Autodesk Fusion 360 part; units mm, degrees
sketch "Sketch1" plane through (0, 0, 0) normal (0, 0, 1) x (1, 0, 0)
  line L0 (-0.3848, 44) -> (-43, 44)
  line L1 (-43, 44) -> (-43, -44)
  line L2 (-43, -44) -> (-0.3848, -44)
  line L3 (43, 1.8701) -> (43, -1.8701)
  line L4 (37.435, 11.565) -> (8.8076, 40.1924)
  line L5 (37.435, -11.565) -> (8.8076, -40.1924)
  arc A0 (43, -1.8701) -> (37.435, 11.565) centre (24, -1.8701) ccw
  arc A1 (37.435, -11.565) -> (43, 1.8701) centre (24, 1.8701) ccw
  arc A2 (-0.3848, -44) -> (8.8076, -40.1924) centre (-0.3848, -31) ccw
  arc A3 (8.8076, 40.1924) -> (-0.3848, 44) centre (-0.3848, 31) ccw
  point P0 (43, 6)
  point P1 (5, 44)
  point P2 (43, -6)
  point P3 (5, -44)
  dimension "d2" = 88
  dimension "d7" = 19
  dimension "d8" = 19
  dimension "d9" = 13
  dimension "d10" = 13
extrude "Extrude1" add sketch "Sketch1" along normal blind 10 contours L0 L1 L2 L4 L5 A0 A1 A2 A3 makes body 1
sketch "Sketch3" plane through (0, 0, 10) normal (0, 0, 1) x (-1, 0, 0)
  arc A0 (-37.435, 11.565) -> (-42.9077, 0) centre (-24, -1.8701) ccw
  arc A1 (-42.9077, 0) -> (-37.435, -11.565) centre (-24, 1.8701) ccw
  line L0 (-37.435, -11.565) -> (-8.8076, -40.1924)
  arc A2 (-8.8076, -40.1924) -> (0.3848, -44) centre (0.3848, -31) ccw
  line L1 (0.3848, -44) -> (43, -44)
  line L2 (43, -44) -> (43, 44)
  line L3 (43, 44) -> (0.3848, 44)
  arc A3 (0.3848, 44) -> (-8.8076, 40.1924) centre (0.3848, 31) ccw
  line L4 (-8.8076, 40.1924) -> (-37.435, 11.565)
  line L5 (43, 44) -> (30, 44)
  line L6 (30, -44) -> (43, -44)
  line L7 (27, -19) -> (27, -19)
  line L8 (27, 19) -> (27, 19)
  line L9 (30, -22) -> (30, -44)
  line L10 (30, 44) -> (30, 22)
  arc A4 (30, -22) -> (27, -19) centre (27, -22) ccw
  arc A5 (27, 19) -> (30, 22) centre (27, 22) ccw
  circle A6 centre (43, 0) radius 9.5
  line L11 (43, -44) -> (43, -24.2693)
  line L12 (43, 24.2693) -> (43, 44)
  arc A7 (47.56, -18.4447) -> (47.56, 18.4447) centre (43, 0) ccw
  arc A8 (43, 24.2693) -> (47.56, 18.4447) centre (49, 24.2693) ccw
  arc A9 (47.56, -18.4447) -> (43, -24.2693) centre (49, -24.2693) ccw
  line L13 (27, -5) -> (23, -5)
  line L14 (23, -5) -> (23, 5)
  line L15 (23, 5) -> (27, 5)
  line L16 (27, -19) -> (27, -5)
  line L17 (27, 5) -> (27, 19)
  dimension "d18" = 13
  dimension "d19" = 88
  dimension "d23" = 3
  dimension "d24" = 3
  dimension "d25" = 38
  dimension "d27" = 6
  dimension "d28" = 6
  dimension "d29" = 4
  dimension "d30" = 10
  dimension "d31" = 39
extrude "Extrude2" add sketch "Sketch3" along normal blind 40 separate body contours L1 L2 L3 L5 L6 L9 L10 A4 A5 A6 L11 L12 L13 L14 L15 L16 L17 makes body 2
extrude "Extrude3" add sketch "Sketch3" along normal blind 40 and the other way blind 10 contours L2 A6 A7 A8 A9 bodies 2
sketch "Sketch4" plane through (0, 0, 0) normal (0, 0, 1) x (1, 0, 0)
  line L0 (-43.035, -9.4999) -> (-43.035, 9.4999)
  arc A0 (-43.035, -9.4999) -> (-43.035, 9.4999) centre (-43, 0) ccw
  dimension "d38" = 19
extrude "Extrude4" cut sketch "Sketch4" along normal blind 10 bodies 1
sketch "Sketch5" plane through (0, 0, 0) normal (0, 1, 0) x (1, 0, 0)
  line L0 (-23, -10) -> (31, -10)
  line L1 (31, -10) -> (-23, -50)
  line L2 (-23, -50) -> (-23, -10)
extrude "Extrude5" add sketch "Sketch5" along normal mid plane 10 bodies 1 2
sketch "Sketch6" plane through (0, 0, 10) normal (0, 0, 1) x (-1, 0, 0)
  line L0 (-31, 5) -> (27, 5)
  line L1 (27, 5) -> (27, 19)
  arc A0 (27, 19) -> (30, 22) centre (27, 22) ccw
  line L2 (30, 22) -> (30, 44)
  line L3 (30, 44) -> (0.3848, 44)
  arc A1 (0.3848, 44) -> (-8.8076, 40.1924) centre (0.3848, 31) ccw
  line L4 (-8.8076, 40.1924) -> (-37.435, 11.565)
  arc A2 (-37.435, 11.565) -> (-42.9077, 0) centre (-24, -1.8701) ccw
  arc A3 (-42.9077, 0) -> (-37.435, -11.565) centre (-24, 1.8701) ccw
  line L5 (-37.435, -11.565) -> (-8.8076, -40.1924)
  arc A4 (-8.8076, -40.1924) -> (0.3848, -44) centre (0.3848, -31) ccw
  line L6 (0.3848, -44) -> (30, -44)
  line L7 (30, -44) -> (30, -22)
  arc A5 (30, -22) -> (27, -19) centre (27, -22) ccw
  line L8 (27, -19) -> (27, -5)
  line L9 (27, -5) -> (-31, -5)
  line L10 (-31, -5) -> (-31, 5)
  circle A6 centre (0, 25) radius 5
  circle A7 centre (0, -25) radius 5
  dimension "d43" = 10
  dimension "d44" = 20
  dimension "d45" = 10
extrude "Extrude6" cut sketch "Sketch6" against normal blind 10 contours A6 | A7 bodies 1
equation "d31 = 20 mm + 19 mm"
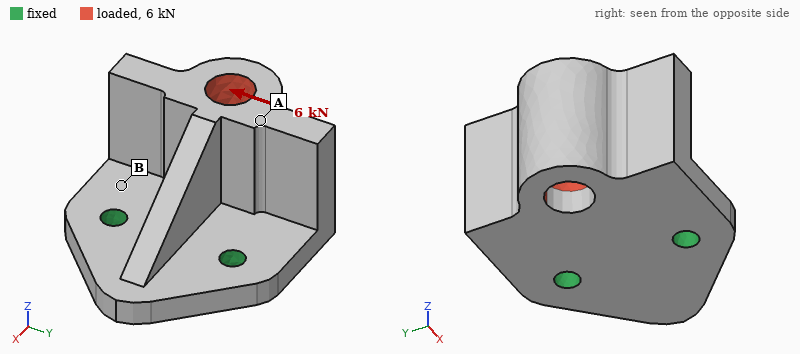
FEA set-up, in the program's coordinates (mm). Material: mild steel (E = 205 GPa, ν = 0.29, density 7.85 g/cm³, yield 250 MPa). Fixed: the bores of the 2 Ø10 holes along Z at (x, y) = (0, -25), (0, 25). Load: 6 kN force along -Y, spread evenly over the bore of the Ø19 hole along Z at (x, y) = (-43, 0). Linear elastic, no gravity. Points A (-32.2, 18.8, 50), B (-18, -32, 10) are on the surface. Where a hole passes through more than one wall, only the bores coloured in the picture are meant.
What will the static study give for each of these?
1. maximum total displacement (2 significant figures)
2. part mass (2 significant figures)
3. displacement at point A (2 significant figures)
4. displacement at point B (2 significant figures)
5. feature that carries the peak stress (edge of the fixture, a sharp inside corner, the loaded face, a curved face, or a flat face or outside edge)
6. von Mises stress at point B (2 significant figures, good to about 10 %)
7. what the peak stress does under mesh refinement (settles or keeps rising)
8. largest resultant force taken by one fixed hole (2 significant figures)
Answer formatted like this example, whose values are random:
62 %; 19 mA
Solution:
30 µm; 1.1 kg; 25 µm; 7.6 µm; edge of the fixture; 23 MPa; keeps rising; 6.0 kN
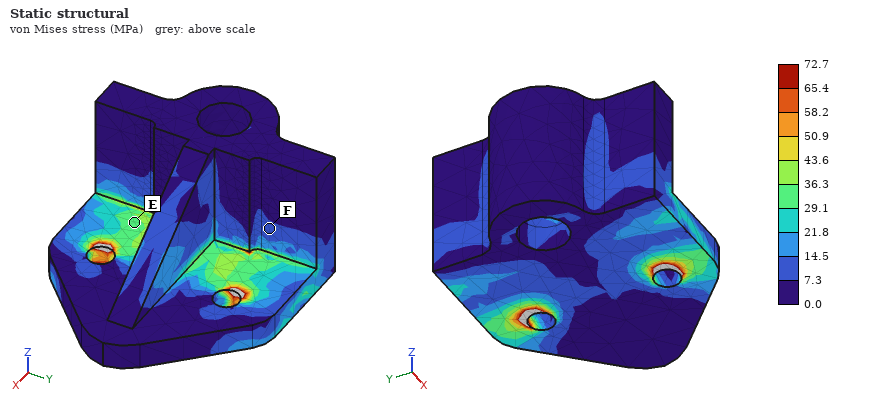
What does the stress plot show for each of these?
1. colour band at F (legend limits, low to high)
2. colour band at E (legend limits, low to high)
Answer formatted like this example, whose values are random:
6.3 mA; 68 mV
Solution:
7.3 to 14.5 MPa; 29.1 to 36.3 MPa
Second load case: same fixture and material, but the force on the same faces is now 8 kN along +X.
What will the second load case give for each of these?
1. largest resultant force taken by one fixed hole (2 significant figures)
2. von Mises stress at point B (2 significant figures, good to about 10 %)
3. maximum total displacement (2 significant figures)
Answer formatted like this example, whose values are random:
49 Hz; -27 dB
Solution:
4.0 kN; 37 MPa; 84 µm
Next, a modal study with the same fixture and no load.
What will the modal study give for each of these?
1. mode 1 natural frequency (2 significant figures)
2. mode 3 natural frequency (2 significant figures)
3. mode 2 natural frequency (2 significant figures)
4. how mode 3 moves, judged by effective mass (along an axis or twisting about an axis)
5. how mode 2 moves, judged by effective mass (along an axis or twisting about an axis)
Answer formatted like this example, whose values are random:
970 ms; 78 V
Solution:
1700 Hz; 6500 Hz; 3100 Hz; along Y; along Y
